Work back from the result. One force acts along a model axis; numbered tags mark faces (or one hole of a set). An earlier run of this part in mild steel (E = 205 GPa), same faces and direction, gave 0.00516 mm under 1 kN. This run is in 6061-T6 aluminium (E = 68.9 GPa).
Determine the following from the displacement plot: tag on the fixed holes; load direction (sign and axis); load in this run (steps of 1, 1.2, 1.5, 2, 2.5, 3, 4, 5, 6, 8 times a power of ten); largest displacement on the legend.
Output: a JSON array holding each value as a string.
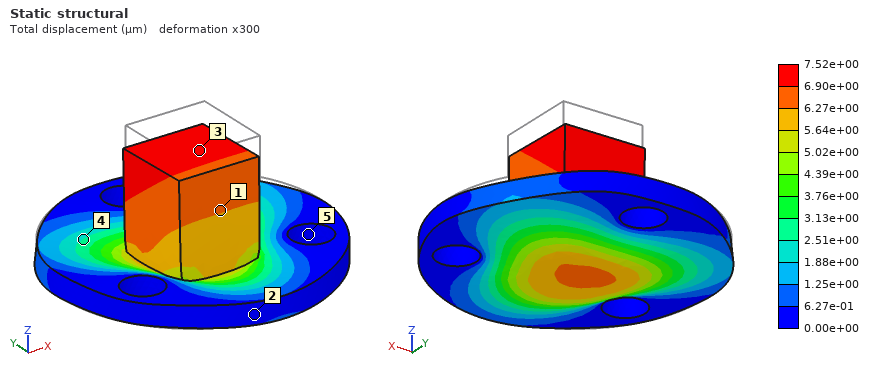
["5", "-Z", "500 N", "7.52e+00 µm"]
